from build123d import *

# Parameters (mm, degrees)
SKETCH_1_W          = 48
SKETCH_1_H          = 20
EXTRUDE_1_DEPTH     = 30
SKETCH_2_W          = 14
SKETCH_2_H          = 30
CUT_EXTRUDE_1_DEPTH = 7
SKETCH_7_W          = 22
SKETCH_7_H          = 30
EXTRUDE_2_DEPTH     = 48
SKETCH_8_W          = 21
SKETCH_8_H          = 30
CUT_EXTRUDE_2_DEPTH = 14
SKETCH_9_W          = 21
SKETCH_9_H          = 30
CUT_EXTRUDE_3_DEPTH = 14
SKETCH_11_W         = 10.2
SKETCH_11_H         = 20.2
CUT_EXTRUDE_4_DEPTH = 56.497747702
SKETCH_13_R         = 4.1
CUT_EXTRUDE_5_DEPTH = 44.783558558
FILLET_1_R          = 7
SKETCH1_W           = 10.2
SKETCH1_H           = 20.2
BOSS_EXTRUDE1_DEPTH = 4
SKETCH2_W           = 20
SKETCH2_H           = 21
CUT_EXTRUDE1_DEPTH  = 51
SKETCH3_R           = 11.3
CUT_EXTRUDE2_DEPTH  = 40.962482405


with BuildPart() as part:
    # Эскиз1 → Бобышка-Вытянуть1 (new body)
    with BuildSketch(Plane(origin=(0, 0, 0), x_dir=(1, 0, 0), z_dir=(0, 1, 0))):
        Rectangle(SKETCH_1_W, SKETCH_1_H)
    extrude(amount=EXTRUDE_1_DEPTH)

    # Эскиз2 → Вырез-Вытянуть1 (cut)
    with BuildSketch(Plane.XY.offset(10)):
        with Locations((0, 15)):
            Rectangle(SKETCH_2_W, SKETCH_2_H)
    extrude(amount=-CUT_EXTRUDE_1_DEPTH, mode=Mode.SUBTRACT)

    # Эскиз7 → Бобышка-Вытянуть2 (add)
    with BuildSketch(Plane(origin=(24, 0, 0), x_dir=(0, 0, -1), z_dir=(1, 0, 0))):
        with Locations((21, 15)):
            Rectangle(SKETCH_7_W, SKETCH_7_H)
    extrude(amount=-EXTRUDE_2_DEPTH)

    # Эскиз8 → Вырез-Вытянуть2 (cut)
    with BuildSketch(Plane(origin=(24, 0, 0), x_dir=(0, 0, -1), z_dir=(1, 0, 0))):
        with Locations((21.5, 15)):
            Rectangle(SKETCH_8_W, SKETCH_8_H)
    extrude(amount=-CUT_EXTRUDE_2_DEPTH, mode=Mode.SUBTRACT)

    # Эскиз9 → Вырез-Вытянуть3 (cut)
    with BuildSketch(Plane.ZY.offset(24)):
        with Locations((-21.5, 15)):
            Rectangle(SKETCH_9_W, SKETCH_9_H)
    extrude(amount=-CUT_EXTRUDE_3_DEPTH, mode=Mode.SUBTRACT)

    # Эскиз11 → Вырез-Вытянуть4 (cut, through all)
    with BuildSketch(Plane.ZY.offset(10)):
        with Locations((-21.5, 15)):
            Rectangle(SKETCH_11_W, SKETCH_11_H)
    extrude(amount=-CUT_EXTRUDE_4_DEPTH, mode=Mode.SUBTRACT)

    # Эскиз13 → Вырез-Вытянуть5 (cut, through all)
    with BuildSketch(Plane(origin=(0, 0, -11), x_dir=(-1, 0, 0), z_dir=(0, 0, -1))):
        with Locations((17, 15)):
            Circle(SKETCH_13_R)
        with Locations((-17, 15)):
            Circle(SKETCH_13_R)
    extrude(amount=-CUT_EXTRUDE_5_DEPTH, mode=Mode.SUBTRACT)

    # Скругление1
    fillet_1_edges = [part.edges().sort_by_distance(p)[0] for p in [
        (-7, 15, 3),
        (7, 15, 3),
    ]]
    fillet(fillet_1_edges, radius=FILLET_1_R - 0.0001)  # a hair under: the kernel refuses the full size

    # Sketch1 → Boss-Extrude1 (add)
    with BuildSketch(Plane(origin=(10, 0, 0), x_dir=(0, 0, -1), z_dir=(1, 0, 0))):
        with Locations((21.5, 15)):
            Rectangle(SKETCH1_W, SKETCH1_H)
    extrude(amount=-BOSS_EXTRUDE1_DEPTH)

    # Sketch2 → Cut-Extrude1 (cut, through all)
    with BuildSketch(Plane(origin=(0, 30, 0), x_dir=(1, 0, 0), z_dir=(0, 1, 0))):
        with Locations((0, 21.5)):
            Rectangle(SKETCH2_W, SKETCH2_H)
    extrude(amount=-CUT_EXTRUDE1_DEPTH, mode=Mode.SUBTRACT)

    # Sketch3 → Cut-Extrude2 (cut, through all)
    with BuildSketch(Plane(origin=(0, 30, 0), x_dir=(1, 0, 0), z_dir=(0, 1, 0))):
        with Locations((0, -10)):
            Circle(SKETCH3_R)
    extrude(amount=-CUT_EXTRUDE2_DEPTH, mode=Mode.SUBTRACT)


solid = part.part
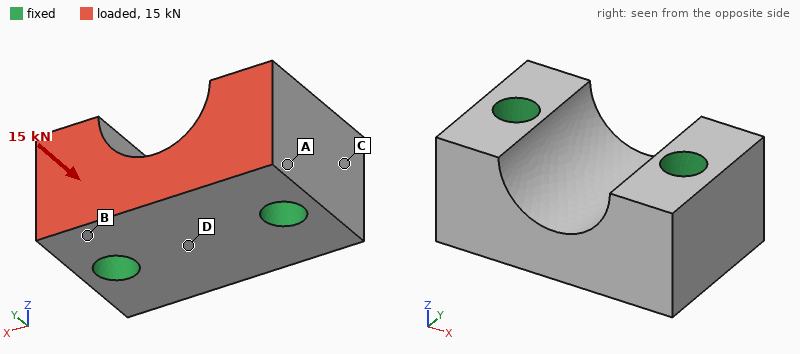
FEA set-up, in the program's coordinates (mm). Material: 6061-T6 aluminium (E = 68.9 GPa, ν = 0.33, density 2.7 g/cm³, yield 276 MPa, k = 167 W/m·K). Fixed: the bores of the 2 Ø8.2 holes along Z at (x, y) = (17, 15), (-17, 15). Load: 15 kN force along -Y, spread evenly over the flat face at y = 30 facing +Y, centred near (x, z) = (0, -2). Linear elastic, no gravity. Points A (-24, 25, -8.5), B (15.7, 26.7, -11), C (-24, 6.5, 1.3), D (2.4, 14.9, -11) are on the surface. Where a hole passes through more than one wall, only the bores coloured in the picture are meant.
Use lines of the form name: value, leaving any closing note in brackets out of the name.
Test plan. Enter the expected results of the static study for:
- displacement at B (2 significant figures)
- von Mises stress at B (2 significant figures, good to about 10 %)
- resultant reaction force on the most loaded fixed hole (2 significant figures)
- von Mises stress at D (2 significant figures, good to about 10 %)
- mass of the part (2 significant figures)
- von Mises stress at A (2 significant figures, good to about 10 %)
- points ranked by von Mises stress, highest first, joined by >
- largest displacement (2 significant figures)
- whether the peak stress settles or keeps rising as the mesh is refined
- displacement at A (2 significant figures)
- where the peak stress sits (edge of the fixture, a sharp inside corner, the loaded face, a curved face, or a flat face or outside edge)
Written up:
displacement at B: 3.3 µm
von Mises stress at B: 20 MPa
resultant reaction force on the most loaded fixed hole: 7.5 kN
von Mises stress at D: 8.7 MPa
mass of the part: 59 g
von Mises stress at A: 15 MPa
points ranked by von Mises stress, highest first, joined by >: B > A > D > C
largest displacement: 7.2 µm
whether the peak stress settles or keeps rising as the mesh is refined: keeps rising
displacement at A: 2.5 µm
where the peak stress sits: edge of the fixture
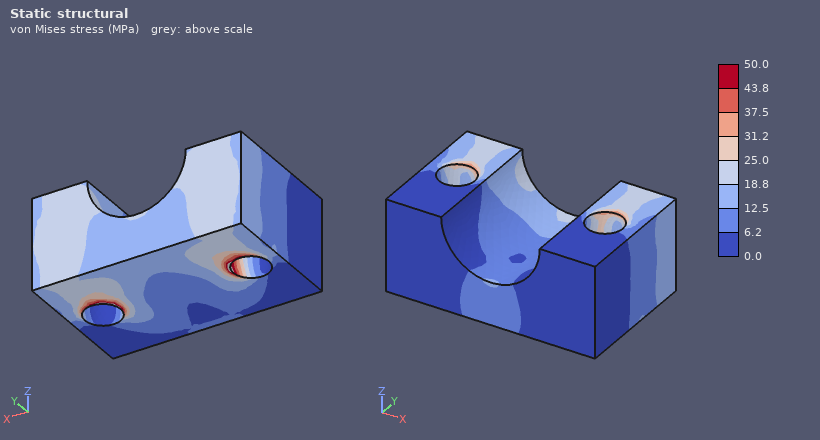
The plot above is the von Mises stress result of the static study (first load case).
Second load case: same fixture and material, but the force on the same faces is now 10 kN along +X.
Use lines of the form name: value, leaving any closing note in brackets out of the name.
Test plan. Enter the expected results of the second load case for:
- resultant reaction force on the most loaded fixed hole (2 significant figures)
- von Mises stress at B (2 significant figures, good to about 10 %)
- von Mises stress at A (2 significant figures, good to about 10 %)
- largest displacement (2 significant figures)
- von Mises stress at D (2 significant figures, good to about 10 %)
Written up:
resultant reaction force on the most loaded fixed hole: 5.6 kN
von Mises stress at B: 26 MPa
von Mises stress at A: 21 MPa
largest displacement: 15 µm
von Mises stress at D: 12 MPa
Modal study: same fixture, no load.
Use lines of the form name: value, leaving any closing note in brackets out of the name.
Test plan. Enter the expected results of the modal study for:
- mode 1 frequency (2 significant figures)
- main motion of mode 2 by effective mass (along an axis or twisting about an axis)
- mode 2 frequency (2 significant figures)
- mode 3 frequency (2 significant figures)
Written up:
mode 1 frequency: 37 kHz
main motion of mode 2 by effective mass: along Z
mode 2 frequency: 39 kHz
mode 3 frequency: 44 kHz
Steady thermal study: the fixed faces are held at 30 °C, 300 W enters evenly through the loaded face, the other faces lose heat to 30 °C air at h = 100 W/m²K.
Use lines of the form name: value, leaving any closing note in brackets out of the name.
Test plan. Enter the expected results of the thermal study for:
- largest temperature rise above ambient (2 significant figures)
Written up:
largest temperature rise above ambient: 34 K
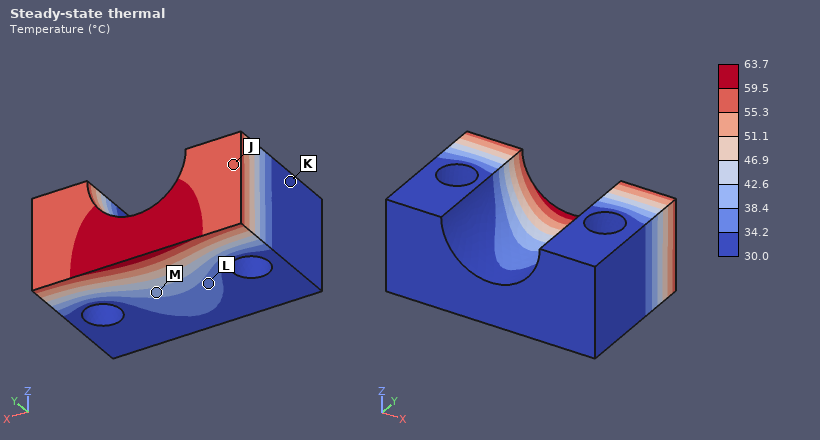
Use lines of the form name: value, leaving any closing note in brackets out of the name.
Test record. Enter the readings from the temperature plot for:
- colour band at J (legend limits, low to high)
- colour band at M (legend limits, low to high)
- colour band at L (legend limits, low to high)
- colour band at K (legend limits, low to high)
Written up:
colour band at J: 55.3 to 59.5 °C
colour band at M: 38.4 to 42.6 °C
colour band at L: 34.2 to 38.4 °C
colour band at K: 30.0 to 34.2 °C
